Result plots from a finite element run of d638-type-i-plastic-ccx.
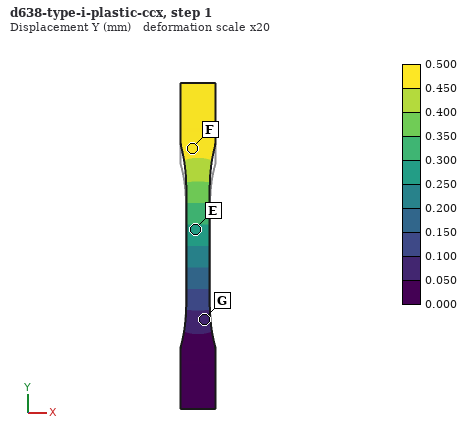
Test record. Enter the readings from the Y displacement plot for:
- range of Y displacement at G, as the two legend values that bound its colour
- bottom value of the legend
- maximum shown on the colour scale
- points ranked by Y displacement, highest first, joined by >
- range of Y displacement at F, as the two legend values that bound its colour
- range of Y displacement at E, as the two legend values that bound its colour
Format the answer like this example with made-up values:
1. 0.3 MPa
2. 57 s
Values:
1. 0.050 to 0.100 mm
2. 0.000 mm
3. 0.500 mm
4. F > E > G
5. 0.450 to 0.500 mm
6. 0.250 to 0.300 mm
